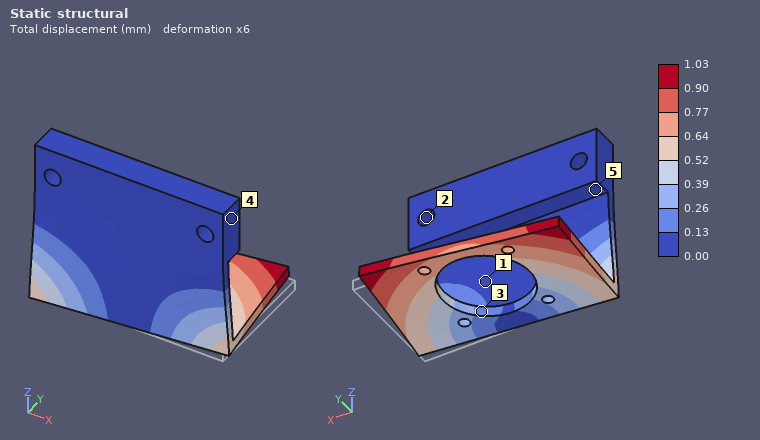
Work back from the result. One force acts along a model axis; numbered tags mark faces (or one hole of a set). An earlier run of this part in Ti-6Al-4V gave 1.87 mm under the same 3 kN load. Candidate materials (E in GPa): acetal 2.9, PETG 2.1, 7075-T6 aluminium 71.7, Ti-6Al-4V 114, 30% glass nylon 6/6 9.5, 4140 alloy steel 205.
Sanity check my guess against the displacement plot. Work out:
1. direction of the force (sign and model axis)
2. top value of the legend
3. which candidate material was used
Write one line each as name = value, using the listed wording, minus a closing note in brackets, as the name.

direction of the force = -X
top value of the legend = 1.03 mm
which candidate material was used = 4140 alloy steel
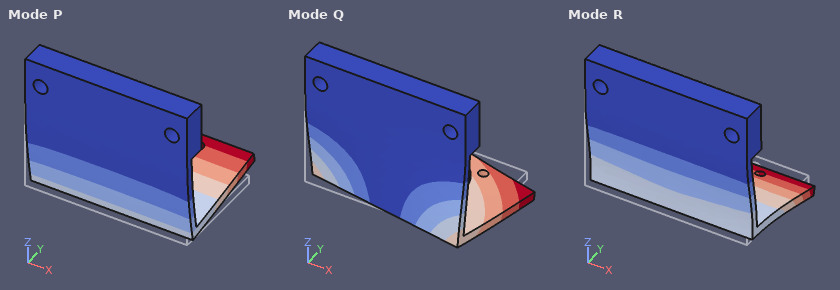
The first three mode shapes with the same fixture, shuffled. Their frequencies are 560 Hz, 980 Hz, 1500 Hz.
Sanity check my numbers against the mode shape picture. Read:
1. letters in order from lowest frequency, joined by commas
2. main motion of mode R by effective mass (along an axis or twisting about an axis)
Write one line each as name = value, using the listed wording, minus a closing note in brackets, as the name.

letters in order from lowest frequency, joined by commas = P, Q, R
main motion of mode R by effective mass = along Y
